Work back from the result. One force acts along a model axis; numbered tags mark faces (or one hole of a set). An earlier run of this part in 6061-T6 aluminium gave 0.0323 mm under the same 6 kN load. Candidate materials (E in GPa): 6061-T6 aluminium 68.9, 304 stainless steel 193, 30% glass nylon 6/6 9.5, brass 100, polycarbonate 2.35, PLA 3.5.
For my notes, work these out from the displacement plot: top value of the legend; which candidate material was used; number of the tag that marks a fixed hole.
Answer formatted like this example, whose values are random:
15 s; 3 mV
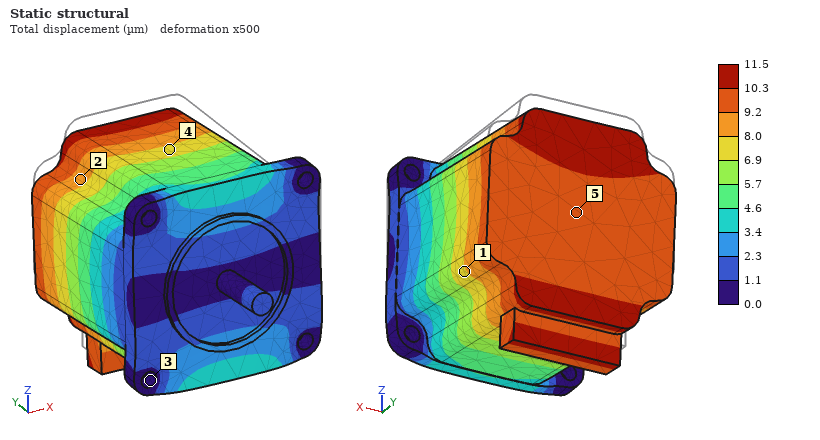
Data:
11.5 µm; 304 stainless steel; 3
